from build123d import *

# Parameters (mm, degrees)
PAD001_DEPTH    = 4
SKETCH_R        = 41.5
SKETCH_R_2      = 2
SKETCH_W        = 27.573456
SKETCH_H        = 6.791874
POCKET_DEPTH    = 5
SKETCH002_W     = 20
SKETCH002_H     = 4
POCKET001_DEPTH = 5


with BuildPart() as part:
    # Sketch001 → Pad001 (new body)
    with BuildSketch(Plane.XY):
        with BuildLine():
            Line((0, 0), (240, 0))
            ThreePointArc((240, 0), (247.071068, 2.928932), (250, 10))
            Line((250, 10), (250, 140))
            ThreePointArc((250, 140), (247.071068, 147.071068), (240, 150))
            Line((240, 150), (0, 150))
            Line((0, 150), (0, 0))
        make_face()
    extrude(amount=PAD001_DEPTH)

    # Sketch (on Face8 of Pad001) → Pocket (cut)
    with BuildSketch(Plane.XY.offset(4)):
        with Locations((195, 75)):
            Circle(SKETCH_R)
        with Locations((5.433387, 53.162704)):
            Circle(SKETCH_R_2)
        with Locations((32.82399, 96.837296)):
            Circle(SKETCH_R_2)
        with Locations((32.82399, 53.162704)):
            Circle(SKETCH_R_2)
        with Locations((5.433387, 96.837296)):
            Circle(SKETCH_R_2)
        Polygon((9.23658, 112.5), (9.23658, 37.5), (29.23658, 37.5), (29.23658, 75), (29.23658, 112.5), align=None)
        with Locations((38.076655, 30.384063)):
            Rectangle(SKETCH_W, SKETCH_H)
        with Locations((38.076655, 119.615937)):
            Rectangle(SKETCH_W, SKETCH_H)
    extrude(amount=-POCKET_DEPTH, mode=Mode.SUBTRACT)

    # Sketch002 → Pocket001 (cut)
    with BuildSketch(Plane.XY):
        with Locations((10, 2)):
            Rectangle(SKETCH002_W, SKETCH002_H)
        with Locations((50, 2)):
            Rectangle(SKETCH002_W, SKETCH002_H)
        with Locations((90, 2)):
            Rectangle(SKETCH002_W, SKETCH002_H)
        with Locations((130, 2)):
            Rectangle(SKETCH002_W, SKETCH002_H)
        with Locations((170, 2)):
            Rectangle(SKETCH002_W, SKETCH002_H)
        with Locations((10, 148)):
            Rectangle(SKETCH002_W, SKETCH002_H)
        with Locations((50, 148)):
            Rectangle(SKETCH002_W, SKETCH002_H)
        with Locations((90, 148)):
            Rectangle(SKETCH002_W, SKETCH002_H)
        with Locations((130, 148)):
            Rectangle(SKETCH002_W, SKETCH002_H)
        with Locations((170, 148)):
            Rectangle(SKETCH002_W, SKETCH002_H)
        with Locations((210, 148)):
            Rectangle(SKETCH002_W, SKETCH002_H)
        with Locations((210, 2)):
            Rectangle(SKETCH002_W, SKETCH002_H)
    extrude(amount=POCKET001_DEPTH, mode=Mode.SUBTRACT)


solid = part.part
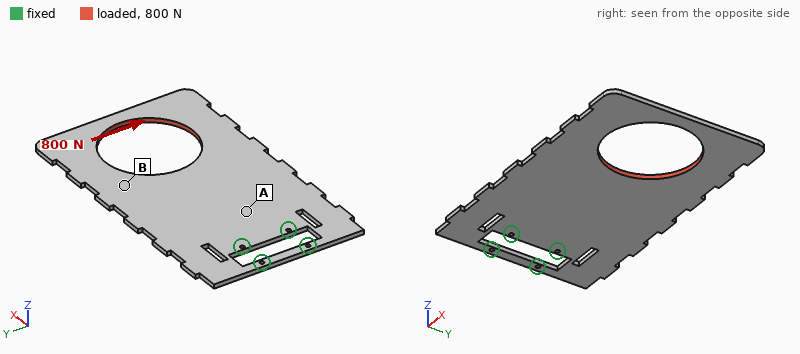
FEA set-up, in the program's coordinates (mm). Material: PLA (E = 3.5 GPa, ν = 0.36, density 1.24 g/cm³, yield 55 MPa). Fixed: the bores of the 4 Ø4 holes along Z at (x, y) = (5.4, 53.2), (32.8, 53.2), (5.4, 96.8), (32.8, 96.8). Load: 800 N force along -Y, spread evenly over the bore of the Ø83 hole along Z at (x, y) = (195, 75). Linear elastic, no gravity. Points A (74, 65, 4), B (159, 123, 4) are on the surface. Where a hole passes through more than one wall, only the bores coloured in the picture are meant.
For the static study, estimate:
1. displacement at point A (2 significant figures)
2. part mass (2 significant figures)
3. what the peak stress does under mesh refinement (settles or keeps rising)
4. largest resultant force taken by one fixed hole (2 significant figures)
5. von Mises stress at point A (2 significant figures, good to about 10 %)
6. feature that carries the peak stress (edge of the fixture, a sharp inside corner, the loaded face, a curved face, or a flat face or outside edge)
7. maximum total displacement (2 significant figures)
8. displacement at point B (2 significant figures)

0.52 mm
140 g
keeps rising
2.2 kN
8.5 MPa
edge of the fixture
3.4 mm
1.8 mm
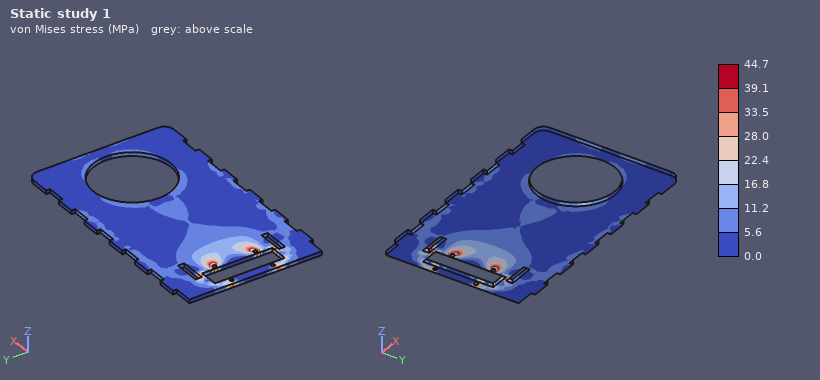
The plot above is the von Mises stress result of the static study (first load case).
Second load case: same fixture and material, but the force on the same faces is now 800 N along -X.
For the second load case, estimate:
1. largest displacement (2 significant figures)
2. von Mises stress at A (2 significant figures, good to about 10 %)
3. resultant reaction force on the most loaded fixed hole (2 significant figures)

0.26 mm
1.7 MPa
380 N
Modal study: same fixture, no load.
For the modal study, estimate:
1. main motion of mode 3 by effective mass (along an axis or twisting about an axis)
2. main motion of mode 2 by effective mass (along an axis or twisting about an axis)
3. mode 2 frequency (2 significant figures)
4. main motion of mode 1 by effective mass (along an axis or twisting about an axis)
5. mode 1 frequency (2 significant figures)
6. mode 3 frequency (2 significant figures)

along Z
twisting about X
64 Hz
along Z
25 Hz
120 Hz
